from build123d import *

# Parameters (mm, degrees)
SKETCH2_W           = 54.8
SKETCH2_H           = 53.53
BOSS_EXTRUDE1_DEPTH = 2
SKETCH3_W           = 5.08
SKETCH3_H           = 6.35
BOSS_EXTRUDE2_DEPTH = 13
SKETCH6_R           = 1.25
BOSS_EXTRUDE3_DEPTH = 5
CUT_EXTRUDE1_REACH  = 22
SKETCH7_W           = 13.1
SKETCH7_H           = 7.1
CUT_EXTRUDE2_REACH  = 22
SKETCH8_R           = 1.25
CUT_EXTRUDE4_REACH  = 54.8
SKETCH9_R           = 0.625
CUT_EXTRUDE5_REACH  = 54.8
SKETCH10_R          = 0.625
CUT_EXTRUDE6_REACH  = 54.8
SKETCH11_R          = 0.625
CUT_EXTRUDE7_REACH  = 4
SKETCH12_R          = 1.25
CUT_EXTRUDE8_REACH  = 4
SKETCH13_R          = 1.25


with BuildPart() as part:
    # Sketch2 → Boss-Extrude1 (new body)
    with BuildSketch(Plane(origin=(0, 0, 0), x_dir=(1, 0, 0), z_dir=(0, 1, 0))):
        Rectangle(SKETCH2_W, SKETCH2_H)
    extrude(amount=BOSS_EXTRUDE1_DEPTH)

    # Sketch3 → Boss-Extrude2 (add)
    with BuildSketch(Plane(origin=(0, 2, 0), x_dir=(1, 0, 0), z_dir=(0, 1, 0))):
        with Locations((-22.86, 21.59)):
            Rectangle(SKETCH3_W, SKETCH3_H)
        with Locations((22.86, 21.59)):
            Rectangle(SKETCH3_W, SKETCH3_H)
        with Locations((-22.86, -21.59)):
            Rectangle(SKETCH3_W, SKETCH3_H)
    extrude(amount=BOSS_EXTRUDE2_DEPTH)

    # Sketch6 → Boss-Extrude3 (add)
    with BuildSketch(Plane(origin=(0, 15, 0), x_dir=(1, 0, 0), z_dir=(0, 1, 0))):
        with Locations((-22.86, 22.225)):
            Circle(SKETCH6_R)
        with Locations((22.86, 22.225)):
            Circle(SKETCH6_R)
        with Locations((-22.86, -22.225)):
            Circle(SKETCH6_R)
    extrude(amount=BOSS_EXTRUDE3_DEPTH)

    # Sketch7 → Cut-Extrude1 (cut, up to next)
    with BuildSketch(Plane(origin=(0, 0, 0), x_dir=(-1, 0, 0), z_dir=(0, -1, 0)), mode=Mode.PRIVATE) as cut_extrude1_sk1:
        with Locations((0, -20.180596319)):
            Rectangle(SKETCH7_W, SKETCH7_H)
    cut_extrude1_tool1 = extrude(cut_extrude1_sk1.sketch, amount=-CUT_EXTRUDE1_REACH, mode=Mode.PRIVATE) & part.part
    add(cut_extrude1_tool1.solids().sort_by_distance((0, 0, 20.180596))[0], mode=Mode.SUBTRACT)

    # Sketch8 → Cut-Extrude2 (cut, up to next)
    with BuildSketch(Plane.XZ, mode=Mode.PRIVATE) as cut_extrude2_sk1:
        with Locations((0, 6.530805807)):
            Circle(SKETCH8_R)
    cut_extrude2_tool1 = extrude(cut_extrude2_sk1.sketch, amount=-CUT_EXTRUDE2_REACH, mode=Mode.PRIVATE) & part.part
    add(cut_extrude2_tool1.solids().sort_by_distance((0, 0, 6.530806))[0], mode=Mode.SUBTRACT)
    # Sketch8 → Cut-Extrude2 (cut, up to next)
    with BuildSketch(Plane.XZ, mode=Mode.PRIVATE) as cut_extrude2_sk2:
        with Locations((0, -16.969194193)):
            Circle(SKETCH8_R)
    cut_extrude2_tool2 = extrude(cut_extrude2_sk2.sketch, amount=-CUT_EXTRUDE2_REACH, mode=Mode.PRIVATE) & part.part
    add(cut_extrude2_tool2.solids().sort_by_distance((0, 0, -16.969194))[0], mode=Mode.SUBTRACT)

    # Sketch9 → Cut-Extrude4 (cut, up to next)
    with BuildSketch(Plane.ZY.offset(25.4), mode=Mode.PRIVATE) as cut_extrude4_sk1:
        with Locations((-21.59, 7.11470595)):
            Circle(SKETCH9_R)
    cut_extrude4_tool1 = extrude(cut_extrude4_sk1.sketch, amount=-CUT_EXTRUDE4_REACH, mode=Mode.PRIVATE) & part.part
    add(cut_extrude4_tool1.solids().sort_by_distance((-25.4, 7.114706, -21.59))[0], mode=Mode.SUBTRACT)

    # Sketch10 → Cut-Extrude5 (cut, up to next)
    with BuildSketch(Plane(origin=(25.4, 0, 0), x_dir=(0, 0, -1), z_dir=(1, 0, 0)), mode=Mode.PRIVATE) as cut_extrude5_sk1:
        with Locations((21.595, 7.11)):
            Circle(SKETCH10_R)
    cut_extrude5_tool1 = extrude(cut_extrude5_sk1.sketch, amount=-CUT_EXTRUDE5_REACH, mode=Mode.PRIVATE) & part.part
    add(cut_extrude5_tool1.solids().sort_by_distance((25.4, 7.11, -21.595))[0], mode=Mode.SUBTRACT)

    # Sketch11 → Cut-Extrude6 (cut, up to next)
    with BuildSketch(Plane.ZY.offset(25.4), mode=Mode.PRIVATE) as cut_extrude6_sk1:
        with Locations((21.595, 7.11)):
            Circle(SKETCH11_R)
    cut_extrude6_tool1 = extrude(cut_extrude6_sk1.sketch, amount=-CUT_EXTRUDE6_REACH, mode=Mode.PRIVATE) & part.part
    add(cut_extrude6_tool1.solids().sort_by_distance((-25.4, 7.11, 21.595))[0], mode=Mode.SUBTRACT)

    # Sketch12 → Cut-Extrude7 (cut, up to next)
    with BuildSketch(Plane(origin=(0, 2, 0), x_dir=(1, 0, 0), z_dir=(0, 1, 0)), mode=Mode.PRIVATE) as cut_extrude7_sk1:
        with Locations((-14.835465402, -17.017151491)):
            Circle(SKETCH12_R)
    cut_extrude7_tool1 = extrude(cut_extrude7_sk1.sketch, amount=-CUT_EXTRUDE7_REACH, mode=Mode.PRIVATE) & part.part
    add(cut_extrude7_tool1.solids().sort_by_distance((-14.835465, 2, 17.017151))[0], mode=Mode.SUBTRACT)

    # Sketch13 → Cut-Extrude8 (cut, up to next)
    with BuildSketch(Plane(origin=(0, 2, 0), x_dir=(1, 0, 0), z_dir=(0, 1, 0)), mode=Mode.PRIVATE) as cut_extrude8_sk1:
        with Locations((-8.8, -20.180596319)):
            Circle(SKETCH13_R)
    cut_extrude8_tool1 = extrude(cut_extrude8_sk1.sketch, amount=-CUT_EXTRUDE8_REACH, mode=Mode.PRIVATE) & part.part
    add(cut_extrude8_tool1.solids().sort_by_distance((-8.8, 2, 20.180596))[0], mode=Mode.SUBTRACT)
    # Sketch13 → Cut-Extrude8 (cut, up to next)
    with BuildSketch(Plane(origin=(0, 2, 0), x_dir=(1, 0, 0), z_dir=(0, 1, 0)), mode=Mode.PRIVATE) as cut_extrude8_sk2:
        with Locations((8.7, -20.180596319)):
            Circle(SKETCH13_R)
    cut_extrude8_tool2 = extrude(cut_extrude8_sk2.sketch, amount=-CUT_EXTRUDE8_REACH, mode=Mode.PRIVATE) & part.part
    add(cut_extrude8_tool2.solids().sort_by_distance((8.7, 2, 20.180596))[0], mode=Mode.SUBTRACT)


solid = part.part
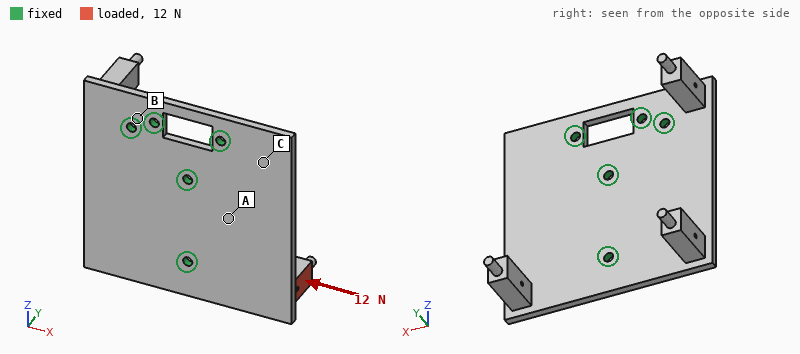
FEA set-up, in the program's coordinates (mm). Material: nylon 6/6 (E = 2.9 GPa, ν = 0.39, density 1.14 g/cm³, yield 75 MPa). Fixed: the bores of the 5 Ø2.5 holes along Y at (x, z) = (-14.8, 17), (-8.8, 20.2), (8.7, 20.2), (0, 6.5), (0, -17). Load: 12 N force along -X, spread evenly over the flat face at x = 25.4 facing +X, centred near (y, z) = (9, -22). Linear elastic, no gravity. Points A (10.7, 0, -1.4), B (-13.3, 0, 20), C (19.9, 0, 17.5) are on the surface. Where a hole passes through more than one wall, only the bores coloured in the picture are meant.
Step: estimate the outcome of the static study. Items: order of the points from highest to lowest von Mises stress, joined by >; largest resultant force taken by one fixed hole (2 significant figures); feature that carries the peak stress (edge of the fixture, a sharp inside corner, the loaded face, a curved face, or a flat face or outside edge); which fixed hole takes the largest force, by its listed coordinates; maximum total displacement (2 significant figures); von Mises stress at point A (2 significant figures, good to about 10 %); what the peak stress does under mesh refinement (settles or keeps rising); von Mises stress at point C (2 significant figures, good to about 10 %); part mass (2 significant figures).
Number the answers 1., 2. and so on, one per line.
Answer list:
1. A > C > B
2. 12 N
3. edge of the fixture
4. (0, -17)
5. 0.80 mm
6. 2.2 MPa
7. keeps rising
8. 1.3 MPa
9. 7.9 g
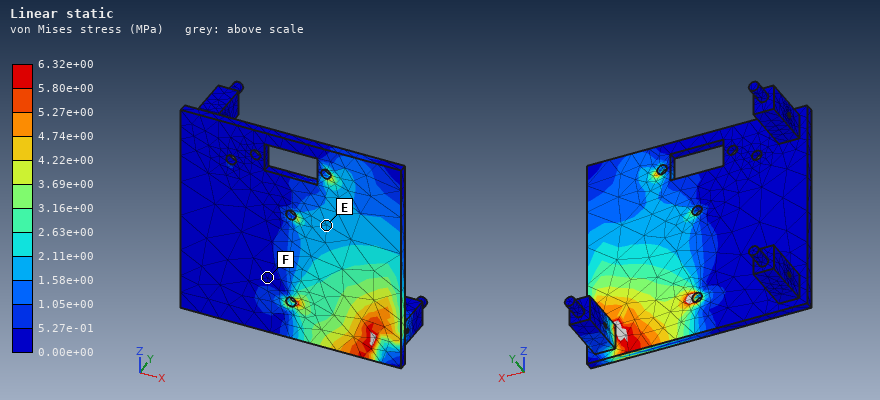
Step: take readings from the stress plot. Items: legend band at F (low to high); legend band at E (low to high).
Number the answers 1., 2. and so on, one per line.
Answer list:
1. 0.00e+00 to 5.27e-01 MPa
2. 1.58e+00 to 2.11e+00 MPa
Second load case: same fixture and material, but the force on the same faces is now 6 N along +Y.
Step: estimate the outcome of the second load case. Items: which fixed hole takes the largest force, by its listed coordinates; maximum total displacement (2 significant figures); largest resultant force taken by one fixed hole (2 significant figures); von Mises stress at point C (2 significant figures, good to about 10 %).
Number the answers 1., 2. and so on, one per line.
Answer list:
1. (0, -17)
2. 0.82 mm
3. 6.2 N
4. 1.4 MPa
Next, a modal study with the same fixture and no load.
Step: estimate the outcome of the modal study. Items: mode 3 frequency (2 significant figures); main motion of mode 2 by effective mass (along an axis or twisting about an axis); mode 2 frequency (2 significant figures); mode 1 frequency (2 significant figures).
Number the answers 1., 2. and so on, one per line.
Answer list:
1. 1100 Hz
2. along Y
3. 600 Hz
4. 530 Hz
